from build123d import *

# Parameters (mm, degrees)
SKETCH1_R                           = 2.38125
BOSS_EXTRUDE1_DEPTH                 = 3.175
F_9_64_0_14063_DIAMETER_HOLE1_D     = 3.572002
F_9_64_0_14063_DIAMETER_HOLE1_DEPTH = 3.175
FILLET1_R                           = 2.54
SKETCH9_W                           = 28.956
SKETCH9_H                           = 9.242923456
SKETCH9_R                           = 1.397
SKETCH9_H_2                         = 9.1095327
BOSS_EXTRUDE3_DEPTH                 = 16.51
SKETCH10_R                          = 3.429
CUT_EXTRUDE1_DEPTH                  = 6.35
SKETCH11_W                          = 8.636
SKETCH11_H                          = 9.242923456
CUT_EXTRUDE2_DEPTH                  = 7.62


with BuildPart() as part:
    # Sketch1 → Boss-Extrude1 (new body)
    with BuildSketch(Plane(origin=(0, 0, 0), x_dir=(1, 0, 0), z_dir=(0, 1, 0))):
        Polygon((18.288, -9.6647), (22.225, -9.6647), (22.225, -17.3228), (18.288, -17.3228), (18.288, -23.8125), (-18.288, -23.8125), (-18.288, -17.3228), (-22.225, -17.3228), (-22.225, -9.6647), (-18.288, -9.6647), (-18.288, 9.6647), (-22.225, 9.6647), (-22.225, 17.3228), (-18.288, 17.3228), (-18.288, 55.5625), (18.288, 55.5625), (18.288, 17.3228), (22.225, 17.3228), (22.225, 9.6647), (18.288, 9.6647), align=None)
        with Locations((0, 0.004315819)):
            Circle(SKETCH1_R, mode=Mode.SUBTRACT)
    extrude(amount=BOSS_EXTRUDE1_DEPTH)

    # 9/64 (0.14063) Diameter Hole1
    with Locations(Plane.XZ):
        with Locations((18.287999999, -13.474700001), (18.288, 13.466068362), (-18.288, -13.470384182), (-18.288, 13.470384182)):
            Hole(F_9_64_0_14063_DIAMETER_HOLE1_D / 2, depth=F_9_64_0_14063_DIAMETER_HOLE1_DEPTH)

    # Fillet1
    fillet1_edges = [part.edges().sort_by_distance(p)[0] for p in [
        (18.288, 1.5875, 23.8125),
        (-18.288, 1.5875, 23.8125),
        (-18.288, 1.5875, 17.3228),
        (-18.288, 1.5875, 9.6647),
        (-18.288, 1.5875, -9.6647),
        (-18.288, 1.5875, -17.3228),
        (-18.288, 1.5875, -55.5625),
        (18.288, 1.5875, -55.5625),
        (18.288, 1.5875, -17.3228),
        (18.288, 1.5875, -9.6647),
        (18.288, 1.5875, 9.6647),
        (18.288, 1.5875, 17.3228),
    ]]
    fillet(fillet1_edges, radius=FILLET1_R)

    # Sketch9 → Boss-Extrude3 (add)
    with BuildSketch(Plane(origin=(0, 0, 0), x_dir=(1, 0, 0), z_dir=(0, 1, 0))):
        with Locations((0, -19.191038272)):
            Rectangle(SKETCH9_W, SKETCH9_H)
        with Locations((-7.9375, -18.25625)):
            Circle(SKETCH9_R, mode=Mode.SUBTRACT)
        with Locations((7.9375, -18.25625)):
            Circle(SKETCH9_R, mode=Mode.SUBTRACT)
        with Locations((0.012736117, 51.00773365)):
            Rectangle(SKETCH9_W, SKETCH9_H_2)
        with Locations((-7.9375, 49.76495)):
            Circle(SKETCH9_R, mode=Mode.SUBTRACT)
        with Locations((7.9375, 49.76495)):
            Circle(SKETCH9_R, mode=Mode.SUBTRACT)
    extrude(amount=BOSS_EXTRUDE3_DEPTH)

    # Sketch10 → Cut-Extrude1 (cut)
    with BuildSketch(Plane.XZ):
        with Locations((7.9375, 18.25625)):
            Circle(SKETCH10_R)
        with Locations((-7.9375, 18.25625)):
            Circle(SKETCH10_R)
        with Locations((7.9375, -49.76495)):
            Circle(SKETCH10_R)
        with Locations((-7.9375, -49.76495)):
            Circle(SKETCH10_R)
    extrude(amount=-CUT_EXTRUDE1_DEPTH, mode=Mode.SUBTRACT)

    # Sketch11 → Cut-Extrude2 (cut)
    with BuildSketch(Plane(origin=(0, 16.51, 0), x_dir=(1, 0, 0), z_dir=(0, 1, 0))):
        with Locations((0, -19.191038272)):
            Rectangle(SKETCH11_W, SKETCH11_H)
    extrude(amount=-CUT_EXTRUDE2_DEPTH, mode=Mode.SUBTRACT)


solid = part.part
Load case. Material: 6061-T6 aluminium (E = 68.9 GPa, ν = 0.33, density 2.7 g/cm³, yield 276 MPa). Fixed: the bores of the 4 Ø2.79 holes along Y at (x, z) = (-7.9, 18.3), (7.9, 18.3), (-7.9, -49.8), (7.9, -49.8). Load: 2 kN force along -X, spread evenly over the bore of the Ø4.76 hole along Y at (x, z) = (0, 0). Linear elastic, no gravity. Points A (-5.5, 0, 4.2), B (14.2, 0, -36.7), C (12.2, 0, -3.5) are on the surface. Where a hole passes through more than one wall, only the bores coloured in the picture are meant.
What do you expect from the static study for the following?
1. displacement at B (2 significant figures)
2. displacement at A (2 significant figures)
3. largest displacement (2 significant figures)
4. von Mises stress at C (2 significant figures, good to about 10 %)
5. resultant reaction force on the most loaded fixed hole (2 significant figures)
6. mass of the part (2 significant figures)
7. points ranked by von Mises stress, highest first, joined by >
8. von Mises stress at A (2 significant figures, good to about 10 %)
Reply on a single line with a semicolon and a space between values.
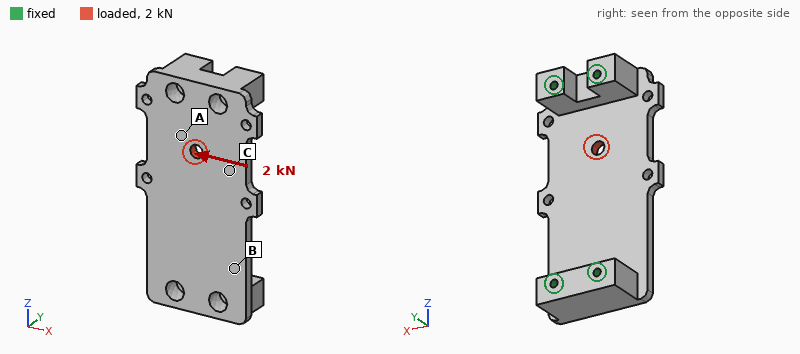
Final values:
9.3 µm; 17 µm; 23 µm; 19 MPa; 950 N; 40 g; A > C > B; 32 MPa
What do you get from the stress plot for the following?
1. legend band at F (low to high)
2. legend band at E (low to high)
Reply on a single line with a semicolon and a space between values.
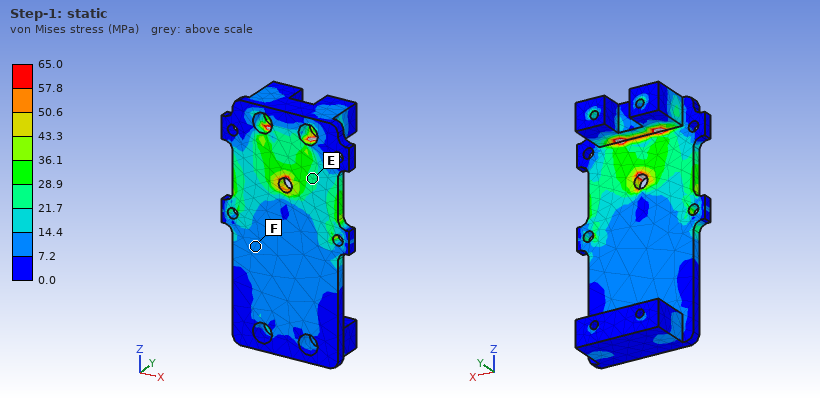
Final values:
7.2 to 14.4 MPa; 21.7 to 28.9 MPa
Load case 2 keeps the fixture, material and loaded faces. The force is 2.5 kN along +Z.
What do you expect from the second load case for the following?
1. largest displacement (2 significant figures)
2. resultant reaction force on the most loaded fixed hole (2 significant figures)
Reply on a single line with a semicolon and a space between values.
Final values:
21 µm; 730 N
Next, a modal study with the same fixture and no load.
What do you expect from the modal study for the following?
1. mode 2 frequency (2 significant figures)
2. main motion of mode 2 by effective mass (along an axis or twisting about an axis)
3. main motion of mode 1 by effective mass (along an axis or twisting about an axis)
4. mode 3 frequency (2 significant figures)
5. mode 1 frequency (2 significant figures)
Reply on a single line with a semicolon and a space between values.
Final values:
5100 Hz; twisting about Z; along Y; 9400 Hz; 3600 Hz
